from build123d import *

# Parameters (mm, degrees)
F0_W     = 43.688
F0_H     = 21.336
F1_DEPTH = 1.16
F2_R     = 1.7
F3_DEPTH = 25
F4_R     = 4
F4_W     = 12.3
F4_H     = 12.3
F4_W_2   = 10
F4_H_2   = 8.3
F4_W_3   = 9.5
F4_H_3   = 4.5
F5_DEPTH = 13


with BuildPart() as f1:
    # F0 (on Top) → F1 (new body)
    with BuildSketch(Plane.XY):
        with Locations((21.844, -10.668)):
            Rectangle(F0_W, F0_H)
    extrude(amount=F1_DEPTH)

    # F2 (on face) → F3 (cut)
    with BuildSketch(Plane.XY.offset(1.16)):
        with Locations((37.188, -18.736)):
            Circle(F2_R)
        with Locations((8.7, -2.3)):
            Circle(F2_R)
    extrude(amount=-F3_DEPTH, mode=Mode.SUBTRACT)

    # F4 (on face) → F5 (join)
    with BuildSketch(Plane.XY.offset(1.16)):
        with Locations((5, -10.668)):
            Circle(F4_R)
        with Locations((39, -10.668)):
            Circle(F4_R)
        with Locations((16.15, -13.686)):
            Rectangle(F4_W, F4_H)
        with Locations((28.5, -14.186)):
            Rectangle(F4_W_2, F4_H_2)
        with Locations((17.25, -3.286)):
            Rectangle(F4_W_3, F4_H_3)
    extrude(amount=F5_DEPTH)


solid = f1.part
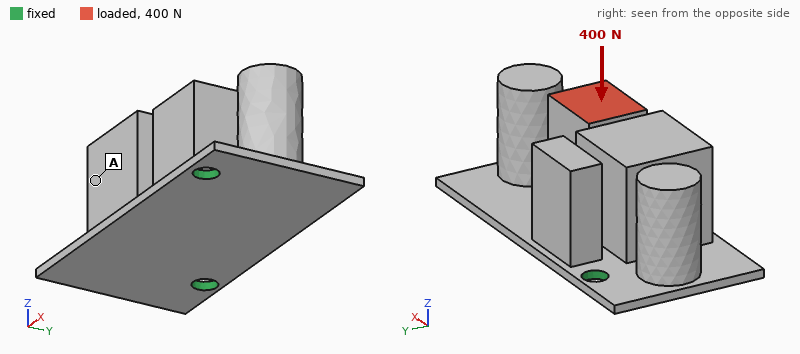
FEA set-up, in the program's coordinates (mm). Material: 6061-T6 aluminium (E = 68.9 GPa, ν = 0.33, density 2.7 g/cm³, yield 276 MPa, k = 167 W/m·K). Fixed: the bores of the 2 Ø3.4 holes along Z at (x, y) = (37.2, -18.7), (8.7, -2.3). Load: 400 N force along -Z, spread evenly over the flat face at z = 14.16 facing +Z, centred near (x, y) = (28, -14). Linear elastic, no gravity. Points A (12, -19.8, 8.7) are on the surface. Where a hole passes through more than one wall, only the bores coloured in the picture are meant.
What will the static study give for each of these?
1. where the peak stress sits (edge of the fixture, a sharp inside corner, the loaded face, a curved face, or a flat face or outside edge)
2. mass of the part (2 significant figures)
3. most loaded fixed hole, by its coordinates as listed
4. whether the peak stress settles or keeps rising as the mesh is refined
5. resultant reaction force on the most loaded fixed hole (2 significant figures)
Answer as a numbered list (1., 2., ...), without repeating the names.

1. edge of the fixture
2. 16 g
3. (37.2, -18.7)
4. keeps rising
5. 320 N
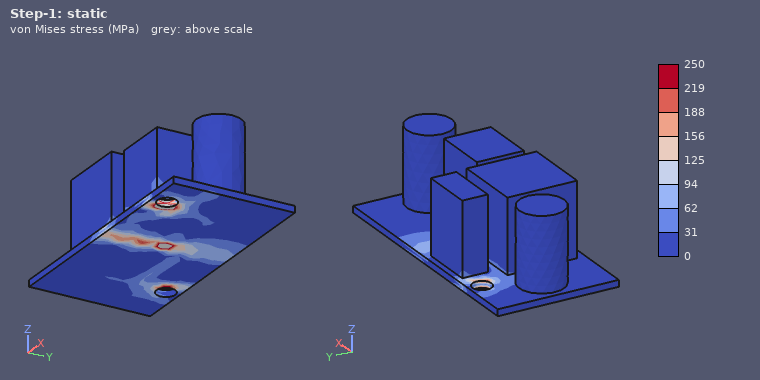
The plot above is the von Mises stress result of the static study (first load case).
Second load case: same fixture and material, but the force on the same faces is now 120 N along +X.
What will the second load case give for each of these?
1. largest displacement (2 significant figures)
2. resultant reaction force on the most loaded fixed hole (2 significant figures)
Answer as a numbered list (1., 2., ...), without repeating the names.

1. 0.16 mm
2. 86 N
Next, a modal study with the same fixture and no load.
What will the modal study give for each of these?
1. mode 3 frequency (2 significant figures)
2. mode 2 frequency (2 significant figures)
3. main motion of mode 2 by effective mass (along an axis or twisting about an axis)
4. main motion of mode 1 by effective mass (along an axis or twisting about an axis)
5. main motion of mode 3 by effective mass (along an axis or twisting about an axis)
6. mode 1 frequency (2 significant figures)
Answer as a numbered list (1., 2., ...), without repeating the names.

1. 3200 Hz
2. 2700 Hz
3. along Z
4. along Y
5. along Z
6. 1500 Hz
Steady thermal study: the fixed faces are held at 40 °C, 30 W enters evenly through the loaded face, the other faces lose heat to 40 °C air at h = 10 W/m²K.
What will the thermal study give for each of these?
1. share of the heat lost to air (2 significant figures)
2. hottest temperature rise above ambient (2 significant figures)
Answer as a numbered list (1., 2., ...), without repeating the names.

1. 3.7 %
2. 71 K
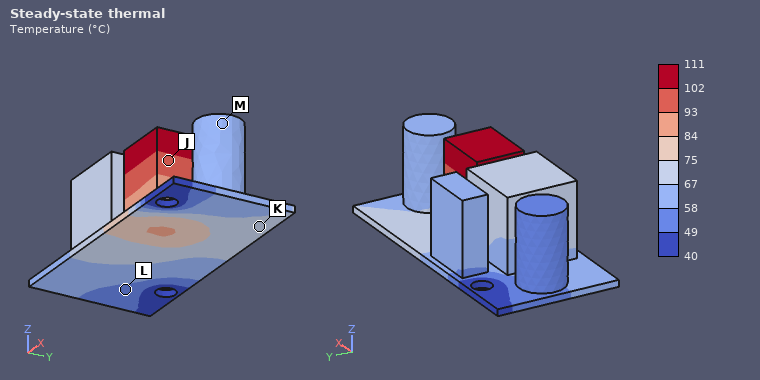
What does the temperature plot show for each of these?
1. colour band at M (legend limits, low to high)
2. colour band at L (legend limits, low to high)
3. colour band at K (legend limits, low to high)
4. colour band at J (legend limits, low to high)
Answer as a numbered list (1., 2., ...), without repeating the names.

1. 58 to 67 °C
2. 49 to 58 °C
3. 67 to 75 °C
4. 93 to 102 °C
